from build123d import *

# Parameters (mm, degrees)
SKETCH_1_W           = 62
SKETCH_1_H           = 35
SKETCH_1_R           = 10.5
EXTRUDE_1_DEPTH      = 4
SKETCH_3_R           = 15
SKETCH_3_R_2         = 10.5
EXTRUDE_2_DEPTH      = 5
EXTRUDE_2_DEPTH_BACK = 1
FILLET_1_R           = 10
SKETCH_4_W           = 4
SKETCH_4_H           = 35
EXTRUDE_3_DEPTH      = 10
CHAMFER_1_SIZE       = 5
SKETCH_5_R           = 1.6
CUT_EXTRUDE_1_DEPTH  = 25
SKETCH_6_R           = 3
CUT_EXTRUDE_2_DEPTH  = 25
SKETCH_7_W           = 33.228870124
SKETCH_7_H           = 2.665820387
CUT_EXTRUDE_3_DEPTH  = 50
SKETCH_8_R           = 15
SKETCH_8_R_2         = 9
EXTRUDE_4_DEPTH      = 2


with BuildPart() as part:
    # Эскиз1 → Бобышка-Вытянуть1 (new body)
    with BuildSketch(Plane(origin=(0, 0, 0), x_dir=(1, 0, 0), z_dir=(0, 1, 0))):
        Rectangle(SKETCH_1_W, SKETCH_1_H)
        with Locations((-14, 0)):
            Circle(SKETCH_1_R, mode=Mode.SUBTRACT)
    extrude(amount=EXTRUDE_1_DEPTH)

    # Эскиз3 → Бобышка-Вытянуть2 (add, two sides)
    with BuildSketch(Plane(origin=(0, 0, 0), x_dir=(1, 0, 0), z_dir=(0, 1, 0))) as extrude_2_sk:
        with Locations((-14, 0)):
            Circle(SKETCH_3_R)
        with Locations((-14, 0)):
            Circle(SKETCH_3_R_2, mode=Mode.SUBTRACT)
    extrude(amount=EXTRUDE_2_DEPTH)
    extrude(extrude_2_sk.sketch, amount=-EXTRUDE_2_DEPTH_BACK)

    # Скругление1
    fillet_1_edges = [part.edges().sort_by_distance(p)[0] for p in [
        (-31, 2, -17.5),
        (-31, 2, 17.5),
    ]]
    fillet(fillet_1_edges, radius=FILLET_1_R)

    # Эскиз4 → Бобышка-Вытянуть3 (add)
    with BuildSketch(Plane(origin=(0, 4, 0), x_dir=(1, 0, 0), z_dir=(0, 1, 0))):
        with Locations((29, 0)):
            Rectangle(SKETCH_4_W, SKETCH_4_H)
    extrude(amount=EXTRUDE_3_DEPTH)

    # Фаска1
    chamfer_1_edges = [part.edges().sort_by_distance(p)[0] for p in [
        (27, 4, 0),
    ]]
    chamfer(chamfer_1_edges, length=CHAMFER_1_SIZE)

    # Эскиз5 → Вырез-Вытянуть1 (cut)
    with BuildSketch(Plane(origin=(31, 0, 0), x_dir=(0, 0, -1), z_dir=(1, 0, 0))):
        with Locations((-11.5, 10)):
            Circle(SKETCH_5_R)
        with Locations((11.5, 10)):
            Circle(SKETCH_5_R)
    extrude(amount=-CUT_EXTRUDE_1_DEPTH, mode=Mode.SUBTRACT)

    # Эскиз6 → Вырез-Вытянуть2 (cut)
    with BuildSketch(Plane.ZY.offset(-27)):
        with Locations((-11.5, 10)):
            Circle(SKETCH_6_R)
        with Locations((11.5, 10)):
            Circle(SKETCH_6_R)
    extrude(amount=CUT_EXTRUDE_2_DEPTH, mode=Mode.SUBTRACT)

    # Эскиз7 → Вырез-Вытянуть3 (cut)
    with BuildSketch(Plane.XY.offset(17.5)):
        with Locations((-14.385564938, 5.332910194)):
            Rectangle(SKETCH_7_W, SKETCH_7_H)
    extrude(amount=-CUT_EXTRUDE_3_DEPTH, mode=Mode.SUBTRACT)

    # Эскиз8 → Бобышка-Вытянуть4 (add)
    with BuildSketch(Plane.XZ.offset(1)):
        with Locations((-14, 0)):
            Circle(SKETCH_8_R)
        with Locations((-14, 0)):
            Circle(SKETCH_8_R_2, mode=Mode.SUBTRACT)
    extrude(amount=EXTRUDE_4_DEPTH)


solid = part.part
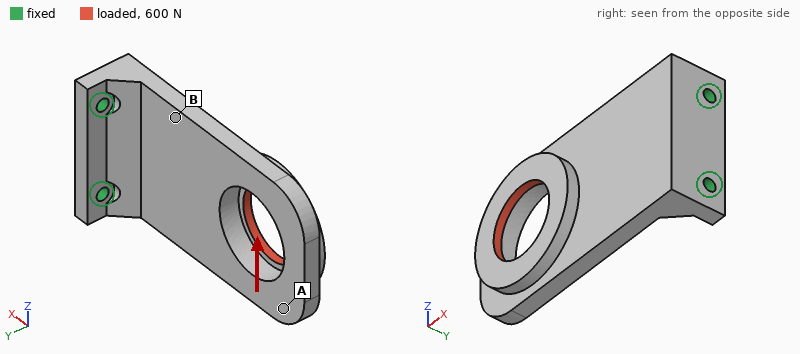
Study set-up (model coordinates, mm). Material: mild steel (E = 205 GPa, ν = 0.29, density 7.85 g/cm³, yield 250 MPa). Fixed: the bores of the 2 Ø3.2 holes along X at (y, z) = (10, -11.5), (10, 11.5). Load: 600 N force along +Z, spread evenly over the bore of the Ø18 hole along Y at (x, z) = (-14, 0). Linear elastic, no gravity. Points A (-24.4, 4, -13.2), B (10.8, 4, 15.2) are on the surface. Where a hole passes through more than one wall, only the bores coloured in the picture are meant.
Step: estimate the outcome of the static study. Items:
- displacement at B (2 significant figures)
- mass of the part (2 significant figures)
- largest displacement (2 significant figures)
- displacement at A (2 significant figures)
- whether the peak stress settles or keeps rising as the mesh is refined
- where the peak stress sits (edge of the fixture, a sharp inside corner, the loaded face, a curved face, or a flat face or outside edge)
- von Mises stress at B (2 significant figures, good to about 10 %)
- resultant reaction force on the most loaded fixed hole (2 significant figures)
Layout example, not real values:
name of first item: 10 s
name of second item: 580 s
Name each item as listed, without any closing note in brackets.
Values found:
displacement at B: 11 µm
mass of the part: 80 g
largest displacement: 34 µm
displacement at A: 30 µm
whether the peak stress settles or keeps rising as the mesh is refined: keeps rising
where the peak stress sits: edge of the fixture
von Mises stress at B: 25 MPa
resultant reaction force on the most loaded fixed hole: 1.1 kN
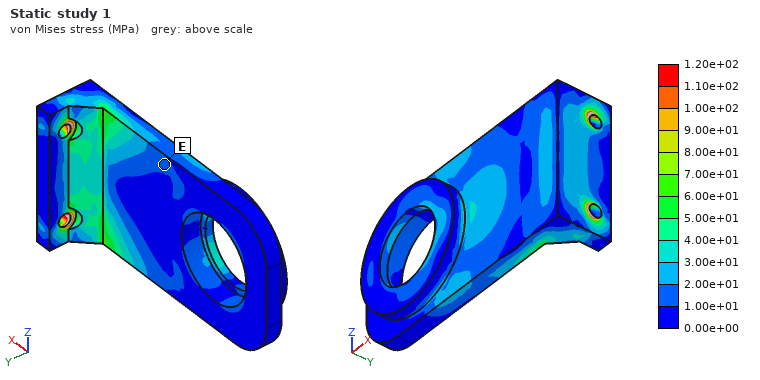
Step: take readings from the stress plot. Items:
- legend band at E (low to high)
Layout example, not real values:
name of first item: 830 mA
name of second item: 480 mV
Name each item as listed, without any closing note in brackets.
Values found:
legend band at E: 1.00e+01 to 2.00e+01 MPa
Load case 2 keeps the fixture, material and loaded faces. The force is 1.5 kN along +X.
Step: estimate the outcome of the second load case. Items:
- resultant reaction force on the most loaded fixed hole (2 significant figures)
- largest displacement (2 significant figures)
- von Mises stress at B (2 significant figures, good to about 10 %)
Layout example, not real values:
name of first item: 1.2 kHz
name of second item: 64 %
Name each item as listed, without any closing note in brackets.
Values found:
resultant reaction force on the most loaded fixed hole: 750 N
largest displacement: 0.31 mm
von Mises stress at B: 51 MPa
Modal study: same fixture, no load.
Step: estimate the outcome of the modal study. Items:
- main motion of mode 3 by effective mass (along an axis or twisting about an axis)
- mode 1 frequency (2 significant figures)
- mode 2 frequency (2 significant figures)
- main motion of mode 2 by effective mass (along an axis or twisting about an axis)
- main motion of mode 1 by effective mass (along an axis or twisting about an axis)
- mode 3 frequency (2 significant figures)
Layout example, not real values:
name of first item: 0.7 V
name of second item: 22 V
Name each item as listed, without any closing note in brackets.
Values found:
main motion of mode 3 by effective mass: along Z
mode 1 frequency: 940 Hz
mode 2 frequency: 3300 Hz
main motion of mode 2 by effective mass: along Z
main motion of mode 1 by effective mass: along Y
mode 3 frequency: 4300 Hz
